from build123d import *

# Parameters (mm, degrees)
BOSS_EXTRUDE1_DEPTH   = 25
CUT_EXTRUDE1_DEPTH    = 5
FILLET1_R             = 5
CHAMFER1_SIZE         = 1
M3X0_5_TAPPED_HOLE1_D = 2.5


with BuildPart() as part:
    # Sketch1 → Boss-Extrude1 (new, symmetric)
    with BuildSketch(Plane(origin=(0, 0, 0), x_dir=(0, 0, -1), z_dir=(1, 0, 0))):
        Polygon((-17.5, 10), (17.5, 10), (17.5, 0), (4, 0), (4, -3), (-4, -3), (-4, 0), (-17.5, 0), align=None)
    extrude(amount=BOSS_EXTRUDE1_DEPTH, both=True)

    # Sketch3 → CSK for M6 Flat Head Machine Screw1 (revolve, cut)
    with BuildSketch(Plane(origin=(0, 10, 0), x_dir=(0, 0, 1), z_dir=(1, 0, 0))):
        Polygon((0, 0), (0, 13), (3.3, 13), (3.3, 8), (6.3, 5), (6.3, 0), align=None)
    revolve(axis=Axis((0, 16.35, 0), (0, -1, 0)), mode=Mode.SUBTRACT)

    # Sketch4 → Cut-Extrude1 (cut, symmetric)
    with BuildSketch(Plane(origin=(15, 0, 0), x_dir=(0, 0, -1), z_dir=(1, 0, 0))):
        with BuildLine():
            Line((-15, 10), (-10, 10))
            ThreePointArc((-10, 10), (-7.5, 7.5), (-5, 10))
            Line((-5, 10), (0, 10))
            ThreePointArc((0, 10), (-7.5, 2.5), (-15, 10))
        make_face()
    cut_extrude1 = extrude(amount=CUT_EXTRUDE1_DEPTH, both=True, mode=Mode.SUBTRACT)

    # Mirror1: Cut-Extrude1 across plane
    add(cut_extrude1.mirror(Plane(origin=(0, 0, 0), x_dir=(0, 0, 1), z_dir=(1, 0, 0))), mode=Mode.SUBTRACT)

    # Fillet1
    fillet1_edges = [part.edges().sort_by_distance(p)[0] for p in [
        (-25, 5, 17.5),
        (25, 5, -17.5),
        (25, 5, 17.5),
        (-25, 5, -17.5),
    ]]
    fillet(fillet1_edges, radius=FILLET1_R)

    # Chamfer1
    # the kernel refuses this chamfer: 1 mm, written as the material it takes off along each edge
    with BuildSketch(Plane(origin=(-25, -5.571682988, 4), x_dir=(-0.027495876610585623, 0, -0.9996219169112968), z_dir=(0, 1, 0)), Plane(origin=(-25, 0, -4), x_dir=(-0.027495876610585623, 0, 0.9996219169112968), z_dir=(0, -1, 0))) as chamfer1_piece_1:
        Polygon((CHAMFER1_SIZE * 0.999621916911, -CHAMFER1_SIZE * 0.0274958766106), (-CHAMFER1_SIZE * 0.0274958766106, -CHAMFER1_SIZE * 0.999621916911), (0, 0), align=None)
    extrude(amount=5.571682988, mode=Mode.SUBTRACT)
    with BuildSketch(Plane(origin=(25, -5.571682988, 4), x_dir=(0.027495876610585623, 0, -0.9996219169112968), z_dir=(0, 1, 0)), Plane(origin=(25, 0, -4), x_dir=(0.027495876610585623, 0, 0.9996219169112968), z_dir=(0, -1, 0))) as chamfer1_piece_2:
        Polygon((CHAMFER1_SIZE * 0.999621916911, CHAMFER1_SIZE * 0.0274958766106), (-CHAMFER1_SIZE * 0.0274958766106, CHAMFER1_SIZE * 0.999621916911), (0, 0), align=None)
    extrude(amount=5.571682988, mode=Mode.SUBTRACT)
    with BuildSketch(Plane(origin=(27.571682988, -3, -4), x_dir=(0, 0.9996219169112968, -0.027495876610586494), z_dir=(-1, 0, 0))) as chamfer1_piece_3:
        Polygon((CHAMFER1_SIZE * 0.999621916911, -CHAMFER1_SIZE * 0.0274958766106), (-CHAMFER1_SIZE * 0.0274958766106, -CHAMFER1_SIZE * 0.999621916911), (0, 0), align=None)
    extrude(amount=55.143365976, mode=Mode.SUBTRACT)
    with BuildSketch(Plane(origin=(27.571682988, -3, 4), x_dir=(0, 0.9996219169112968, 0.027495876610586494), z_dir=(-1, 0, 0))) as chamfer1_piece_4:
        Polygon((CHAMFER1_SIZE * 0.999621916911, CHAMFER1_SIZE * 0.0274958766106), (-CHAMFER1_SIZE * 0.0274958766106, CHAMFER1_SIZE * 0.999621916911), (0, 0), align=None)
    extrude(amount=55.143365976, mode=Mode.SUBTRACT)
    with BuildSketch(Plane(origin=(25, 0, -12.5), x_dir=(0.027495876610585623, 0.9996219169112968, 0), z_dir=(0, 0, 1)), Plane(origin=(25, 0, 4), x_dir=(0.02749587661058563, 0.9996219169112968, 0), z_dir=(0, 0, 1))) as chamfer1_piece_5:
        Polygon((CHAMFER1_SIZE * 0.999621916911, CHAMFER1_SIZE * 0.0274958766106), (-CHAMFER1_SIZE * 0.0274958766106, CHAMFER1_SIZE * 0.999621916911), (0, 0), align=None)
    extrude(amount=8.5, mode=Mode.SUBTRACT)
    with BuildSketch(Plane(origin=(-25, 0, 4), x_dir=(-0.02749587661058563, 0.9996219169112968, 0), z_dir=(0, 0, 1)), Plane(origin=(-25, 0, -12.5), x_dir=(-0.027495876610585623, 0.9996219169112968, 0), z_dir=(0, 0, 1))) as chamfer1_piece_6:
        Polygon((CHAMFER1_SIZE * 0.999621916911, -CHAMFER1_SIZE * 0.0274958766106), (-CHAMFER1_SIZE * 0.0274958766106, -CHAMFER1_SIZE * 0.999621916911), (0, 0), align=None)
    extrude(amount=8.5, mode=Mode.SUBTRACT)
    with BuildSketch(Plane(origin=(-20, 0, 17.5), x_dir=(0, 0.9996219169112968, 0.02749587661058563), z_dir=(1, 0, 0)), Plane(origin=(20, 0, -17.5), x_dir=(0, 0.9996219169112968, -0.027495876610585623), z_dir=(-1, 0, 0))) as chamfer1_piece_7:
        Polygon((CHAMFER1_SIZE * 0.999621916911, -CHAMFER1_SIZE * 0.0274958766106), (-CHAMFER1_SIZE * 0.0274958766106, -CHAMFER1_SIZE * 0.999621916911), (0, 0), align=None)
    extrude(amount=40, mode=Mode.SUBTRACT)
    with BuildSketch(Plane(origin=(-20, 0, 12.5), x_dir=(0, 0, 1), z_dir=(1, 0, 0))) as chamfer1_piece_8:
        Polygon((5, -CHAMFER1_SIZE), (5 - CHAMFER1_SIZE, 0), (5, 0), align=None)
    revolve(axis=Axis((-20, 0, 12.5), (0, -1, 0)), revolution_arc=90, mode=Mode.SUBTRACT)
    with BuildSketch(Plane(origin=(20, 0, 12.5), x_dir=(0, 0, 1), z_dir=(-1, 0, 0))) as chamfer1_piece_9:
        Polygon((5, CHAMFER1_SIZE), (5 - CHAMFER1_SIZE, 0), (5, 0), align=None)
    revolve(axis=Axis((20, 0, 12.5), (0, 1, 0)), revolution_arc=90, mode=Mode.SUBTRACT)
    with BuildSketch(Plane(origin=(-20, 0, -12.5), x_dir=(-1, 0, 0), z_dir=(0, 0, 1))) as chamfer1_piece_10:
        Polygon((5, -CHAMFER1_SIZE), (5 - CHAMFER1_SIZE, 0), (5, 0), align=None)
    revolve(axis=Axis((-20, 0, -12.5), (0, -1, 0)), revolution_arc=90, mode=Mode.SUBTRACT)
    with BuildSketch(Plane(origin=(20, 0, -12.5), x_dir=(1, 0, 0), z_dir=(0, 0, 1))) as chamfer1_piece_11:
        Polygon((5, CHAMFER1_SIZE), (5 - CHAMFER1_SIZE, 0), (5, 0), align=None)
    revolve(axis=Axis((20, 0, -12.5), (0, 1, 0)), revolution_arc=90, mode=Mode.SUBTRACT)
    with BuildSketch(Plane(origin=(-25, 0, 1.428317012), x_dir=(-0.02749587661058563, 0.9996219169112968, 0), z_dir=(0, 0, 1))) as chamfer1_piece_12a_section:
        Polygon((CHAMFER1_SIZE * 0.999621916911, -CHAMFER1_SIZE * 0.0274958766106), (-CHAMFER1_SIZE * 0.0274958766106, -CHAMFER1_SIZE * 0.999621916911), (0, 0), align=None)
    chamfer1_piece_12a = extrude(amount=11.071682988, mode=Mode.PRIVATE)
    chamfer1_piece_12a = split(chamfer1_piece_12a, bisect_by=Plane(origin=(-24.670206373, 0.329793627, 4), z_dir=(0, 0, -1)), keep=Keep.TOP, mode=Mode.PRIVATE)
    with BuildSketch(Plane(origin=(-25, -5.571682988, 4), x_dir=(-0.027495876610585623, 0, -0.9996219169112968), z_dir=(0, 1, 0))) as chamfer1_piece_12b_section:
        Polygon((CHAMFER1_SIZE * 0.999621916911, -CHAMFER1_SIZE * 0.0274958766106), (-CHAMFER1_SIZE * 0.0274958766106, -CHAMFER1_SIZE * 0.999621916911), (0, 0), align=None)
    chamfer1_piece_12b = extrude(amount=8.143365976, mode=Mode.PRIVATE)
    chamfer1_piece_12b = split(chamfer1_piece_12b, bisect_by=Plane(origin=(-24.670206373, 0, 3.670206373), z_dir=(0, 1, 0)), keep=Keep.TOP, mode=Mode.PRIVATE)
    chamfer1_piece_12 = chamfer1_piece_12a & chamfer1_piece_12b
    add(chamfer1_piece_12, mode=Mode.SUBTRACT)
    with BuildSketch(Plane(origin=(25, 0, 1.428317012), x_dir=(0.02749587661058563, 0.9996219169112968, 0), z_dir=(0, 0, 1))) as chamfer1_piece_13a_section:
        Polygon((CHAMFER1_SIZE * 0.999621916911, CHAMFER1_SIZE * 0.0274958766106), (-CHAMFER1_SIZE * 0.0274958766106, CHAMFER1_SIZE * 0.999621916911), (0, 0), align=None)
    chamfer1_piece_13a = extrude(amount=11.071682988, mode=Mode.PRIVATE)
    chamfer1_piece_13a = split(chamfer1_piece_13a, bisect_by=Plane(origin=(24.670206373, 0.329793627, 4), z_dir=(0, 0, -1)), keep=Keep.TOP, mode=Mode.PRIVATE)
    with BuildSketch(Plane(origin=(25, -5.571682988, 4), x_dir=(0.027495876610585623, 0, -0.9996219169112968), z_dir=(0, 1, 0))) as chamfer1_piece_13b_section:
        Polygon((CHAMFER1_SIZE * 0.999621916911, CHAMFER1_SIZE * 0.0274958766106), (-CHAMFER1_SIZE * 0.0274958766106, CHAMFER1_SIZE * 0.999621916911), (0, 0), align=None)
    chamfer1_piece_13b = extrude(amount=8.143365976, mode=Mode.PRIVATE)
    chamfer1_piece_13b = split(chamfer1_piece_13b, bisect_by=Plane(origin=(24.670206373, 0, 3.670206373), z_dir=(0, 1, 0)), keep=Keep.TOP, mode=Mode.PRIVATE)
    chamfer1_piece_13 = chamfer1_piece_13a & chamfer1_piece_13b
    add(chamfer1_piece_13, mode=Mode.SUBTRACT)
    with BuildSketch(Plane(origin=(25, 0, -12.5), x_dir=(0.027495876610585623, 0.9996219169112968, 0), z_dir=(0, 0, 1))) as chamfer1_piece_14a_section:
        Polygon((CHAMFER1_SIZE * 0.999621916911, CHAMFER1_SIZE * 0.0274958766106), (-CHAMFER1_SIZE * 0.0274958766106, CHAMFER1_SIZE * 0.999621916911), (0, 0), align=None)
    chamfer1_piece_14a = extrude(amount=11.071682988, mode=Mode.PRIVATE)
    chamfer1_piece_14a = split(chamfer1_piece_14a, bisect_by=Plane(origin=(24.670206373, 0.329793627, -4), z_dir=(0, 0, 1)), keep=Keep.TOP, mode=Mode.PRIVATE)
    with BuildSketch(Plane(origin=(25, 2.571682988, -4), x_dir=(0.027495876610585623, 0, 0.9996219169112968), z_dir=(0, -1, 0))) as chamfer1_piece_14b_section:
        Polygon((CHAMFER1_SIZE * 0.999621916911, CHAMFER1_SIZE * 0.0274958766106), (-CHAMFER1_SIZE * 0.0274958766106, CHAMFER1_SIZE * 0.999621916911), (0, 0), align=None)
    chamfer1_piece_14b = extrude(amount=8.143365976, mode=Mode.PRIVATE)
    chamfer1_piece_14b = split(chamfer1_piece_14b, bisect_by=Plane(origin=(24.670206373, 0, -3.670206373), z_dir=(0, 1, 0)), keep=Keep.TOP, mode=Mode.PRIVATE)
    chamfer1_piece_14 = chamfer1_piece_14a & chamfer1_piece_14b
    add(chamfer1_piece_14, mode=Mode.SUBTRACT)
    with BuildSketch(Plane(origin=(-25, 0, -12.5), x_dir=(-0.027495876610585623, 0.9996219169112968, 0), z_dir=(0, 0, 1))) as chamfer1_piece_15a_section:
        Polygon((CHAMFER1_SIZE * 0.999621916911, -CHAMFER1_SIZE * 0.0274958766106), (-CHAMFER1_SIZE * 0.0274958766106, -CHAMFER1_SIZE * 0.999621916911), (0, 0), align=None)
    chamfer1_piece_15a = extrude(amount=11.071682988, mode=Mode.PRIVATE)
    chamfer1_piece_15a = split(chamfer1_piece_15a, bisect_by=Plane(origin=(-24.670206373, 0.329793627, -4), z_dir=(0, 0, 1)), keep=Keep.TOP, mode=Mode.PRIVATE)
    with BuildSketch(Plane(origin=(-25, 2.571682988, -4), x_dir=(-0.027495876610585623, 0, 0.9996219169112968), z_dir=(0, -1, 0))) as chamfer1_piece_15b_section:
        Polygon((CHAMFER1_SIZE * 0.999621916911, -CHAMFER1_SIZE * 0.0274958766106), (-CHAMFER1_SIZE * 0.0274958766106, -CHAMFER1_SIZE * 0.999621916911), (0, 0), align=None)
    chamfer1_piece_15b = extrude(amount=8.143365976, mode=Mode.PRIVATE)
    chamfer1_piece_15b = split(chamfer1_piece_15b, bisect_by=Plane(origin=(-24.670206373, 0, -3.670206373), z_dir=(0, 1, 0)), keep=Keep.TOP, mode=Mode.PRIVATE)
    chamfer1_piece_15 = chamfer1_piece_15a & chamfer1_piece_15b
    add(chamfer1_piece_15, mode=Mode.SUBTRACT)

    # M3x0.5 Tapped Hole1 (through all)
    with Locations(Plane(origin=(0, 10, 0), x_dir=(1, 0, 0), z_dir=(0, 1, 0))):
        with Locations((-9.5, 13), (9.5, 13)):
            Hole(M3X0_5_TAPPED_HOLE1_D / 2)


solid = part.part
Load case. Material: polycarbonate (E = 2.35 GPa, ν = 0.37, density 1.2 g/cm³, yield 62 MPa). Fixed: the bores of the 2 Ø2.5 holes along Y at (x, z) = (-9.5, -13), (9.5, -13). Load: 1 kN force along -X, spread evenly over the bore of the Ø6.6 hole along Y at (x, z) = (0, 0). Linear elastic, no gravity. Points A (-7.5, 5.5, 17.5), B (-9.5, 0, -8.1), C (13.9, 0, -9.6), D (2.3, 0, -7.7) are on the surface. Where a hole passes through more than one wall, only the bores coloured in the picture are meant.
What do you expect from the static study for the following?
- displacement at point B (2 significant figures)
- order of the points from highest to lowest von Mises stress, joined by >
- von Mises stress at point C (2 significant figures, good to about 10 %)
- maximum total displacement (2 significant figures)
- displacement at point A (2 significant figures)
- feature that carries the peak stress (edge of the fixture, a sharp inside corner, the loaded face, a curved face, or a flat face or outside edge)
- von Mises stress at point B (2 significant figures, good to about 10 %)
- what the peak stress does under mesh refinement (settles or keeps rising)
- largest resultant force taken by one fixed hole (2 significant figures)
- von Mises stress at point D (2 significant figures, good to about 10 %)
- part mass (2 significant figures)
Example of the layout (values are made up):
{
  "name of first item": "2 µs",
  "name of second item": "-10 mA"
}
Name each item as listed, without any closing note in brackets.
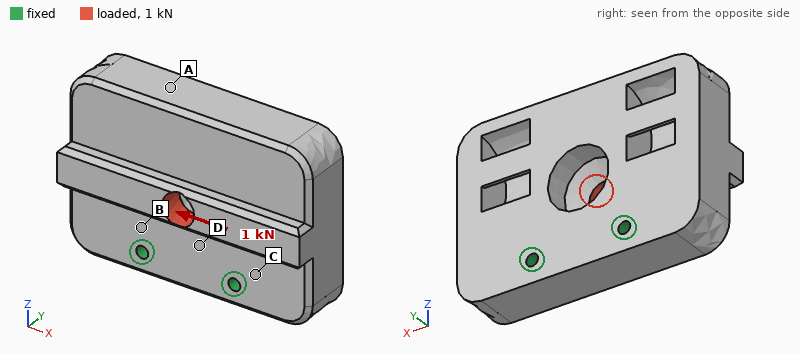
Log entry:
{
  "displacement at point B": "0.048 mm",
  "order of the points from highest to lowest von Mises stress, joined by >": "D > B > C > A",
  "von Mises stress at point C": "5.7 MPa",
  "maximum total displacement": "0.24 mm",
  "displacement at point A": "0.17 mm",
  "feature that carries the peak stress": "a sharp inside corner",
  "von Mises stress at point B": "9.6 MPa",
  "what the peak stress does under mesh refinement": "keeps rising",
  "largest resultant force taken by one fixed hole": "810 N",
  "von Mises stress at point D": "14 MPa",
  "part mass": "19 g"
}
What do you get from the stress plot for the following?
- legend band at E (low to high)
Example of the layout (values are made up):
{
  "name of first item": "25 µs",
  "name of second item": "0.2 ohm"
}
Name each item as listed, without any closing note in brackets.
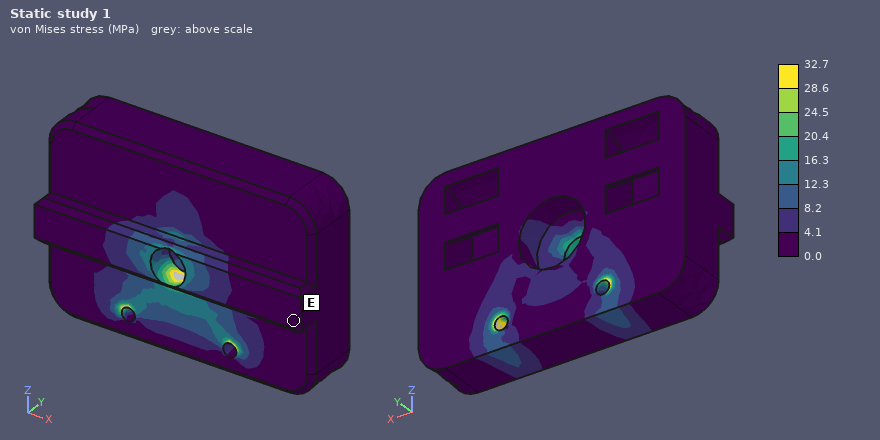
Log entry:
{
  "legend band at E": "0.0 to 4.1 MPa"
}
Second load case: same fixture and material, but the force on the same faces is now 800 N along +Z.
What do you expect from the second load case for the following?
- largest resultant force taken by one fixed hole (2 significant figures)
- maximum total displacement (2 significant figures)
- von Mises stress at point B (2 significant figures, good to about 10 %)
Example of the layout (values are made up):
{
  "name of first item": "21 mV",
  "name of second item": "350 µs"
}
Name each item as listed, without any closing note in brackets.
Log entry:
{
  "largest resultant force taken by one fixed hole": "410 N",
  "maximum total displacement": "0.28 mm",
  "von Mises stress at point B": "13 MPa"
}
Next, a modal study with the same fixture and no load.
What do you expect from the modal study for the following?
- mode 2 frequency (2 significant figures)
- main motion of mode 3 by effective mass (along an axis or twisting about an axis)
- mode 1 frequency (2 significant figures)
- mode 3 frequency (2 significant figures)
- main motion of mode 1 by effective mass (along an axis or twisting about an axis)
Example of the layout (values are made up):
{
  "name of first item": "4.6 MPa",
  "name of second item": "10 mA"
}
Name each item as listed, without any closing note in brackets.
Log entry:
{
  "mode 2 frequency": "2500 Hz",
  "main motion of mode 3 by effective mass": "along X",
  "mode 1 frequency": "1700 Hz",
  "mode 3 frequency": "2900 Hz",
  "main motion of mode 1 by effective mass": "along Y"
}
